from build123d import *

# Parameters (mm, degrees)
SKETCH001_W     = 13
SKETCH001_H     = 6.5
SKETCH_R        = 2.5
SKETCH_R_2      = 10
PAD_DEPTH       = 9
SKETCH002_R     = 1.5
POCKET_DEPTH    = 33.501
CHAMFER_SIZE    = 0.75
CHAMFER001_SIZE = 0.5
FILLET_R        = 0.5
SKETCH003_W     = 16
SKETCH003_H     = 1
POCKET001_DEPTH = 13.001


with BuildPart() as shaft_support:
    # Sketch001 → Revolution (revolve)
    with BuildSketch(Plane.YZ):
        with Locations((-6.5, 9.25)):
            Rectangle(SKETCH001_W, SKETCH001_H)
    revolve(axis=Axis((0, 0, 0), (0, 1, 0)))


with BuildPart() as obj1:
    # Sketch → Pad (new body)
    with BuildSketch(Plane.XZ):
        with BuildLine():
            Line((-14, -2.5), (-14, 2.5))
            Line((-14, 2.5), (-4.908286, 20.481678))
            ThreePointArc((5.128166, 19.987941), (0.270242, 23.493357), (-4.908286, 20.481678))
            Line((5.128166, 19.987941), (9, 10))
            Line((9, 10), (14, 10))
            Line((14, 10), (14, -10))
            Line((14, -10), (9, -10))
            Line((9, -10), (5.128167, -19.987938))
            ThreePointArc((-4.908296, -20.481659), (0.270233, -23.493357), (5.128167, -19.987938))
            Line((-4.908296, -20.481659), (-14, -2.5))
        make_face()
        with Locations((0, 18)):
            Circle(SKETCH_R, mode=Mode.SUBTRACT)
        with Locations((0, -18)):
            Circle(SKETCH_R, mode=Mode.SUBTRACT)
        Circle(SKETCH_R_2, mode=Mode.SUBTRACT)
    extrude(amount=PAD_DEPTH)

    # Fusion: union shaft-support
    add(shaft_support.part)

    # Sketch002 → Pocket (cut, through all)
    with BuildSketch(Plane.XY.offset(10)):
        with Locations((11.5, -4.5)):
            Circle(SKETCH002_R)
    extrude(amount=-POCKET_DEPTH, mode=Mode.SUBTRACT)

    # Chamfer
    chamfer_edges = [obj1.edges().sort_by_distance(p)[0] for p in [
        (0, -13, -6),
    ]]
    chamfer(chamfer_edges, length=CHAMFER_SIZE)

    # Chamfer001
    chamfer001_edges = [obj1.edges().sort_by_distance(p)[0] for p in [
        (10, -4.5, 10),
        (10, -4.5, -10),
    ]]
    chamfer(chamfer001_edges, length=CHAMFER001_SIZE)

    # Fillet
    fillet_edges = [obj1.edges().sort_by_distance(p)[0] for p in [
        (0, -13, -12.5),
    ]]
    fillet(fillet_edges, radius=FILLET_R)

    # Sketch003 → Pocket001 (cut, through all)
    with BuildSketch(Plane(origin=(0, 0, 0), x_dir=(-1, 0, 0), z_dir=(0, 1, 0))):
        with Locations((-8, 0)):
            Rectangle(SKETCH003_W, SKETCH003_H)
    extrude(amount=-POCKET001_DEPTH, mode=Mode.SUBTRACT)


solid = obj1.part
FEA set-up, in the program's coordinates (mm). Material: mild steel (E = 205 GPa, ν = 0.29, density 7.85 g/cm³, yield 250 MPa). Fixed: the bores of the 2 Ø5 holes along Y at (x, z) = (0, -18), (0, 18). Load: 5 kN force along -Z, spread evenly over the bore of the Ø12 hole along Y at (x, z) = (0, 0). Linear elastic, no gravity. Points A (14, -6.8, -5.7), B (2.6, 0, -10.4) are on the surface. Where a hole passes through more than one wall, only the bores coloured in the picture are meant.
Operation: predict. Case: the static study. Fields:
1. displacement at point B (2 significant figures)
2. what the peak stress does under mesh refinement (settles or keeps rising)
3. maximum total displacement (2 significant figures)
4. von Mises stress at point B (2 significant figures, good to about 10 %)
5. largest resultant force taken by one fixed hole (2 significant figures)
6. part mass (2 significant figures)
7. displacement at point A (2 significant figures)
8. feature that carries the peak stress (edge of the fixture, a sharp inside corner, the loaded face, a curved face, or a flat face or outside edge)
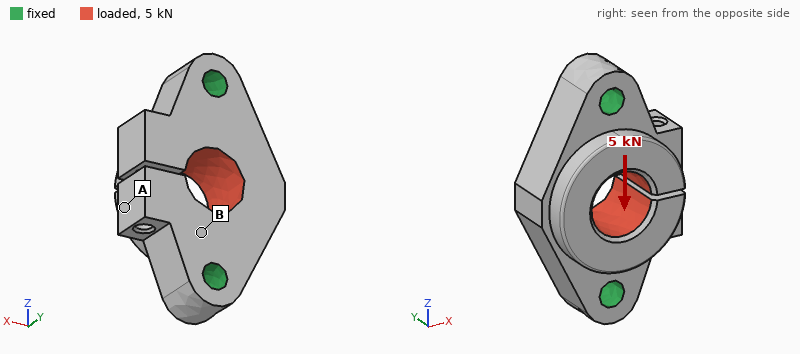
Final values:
0.43 µm
keeps rising
2.7 µm
14 MPa
2.5 kN
61 g
1.4 µm
edge of the fixture
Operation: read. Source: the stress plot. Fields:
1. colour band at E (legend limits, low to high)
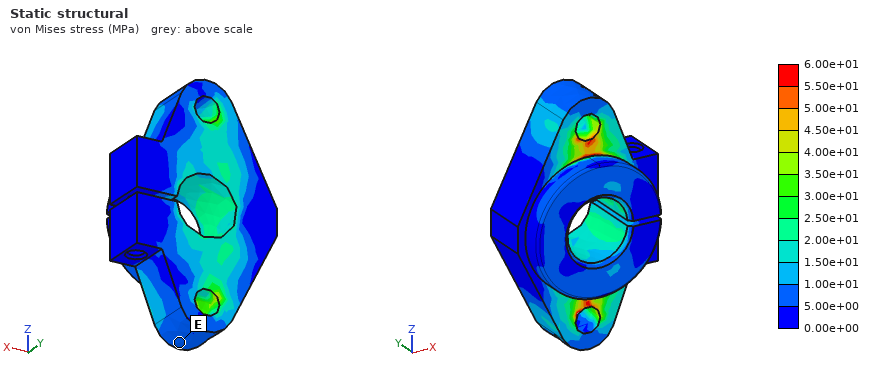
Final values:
5.00e+00 to 1.00e+01 MPa
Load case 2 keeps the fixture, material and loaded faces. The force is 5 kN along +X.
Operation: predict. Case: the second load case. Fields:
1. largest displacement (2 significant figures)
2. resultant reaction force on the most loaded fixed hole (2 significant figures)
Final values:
14 µm
3.2 kN
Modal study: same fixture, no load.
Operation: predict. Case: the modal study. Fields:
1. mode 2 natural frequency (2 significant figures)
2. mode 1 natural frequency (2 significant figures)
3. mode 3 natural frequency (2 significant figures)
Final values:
19 kHz
18 kHz
19 kHz
